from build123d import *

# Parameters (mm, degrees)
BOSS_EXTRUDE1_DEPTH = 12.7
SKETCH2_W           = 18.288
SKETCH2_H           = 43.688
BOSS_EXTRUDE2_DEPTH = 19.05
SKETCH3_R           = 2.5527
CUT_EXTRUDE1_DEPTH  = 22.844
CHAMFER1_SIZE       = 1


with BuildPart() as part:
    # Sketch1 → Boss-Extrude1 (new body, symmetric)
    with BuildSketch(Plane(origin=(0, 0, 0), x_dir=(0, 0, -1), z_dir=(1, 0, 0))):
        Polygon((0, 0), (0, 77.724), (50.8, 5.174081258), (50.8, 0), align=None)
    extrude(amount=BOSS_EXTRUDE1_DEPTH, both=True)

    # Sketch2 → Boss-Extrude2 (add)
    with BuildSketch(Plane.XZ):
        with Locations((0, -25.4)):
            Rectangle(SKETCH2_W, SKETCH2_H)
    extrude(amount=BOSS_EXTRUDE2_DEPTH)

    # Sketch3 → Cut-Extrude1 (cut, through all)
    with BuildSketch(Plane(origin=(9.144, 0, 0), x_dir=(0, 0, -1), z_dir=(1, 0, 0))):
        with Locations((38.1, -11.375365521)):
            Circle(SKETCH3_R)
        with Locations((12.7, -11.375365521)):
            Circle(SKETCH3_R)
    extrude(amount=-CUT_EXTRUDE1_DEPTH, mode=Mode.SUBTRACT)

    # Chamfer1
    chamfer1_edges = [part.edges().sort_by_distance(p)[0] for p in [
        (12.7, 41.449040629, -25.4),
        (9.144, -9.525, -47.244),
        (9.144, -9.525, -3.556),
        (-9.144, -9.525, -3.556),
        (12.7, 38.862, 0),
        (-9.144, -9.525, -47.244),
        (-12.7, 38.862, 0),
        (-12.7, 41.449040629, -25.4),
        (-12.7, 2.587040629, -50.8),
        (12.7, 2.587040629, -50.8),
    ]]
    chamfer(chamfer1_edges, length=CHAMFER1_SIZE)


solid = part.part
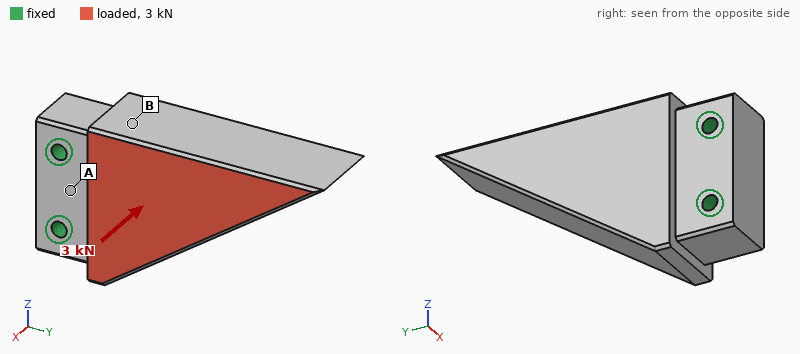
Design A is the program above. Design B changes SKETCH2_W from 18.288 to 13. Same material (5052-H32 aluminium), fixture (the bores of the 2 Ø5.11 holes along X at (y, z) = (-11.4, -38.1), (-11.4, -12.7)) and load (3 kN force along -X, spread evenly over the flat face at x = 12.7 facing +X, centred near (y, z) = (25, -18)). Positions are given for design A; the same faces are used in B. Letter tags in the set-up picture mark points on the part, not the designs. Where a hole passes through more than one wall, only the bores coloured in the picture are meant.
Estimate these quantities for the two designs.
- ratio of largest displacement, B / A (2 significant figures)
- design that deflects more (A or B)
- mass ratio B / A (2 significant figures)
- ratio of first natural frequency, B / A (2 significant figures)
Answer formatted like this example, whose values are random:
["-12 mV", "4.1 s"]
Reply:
["2.2", "B", "0.94", "0.68"]
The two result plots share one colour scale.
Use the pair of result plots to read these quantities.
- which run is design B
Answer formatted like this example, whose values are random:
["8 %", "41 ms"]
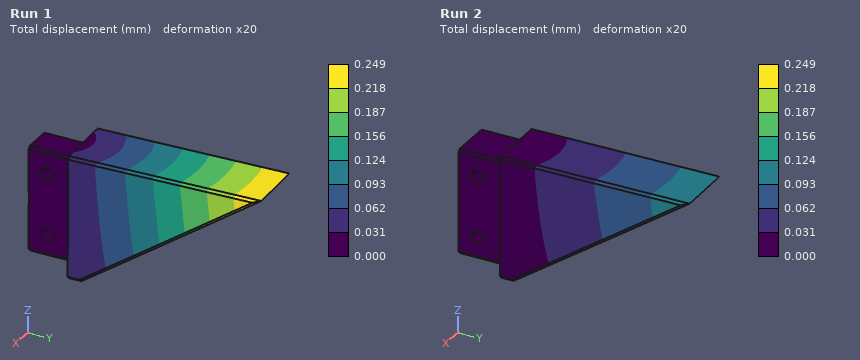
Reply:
["Run 1"]
